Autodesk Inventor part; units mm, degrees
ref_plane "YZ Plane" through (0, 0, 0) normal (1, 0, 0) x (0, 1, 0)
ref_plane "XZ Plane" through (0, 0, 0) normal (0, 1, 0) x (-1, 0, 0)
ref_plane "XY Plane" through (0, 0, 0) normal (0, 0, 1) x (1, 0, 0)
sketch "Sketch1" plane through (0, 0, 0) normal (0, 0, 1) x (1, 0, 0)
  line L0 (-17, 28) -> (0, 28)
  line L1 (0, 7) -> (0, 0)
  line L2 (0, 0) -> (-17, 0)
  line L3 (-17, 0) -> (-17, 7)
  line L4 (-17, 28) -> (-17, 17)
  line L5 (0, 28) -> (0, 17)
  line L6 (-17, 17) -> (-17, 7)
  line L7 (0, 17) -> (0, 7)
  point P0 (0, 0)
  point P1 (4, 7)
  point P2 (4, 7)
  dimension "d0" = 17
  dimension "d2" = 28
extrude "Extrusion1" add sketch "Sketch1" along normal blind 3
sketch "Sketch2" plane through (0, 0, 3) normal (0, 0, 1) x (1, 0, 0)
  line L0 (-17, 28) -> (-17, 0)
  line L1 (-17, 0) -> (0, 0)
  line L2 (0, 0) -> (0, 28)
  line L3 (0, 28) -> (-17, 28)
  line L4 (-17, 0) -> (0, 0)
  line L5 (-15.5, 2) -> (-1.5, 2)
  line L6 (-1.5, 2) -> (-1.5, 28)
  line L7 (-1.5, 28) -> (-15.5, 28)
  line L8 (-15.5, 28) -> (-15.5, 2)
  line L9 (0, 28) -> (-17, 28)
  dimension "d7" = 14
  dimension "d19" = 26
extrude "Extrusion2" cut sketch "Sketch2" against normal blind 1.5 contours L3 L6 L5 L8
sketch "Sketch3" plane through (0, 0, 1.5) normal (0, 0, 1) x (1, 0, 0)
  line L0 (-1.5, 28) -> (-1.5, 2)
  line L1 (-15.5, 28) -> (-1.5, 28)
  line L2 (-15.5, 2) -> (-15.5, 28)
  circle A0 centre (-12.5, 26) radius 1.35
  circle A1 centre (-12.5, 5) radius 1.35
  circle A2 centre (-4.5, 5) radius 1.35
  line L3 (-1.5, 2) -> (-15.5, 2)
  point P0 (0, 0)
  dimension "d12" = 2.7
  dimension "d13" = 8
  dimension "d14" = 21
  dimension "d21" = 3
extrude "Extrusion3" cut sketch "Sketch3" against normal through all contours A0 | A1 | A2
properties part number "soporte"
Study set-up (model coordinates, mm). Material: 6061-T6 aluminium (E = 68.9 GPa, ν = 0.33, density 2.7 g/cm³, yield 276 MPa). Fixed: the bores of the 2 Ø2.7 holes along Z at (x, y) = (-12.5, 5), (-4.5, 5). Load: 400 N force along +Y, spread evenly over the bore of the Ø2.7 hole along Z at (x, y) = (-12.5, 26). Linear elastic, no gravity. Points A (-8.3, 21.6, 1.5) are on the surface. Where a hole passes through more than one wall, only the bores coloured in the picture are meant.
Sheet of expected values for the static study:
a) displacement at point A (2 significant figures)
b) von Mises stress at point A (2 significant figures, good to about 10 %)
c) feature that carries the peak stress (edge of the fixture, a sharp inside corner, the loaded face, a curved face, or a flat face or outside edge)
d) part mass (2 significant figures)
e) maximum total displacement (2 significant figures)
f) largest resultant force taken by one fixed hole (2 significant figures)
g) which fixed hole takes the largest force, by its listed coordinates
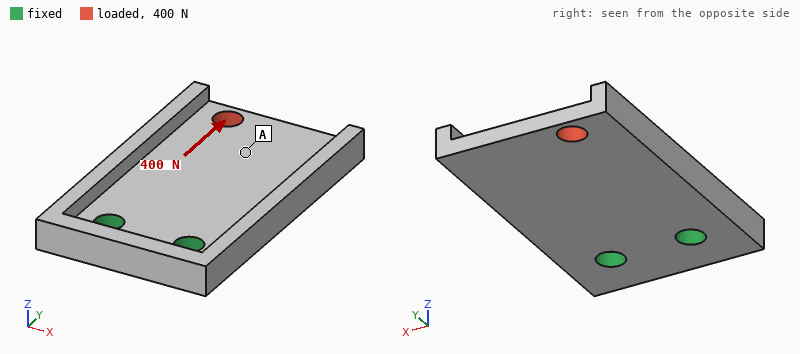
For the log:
10 µm
14 MPa
a flat face or outside edge
2.3 g
26 µm
370 N
(-12.5, 5)
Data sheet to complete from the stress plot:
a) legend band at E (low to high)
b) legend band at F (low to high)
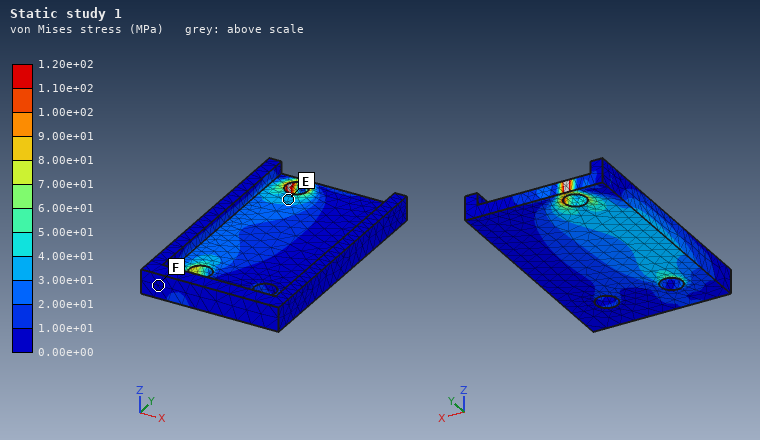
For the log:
3.00e+01 to 4.00e+01 MPa
0.00e+00 to 1.00e+01 MPa
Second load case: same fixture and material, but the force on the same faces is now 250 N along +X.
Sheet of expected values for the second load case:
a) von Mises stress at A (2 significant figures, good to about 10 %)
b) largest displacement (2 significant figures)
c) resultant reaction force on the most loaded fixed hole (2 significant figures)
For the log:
32 MPa
42 µm
530 N
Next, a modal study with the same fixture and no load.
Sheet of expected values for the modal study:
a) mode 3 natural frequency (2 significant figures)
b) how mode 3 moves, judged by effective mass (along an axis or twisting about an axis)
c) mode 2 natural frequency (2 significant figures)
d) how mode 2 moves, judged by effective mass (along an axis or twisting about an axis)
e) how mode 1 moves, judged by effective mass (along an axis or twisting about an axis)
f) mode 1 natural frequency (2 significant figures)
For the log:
17 kHz
along X
7000 Hz
twisting about Y
along Z
3400 Hz
